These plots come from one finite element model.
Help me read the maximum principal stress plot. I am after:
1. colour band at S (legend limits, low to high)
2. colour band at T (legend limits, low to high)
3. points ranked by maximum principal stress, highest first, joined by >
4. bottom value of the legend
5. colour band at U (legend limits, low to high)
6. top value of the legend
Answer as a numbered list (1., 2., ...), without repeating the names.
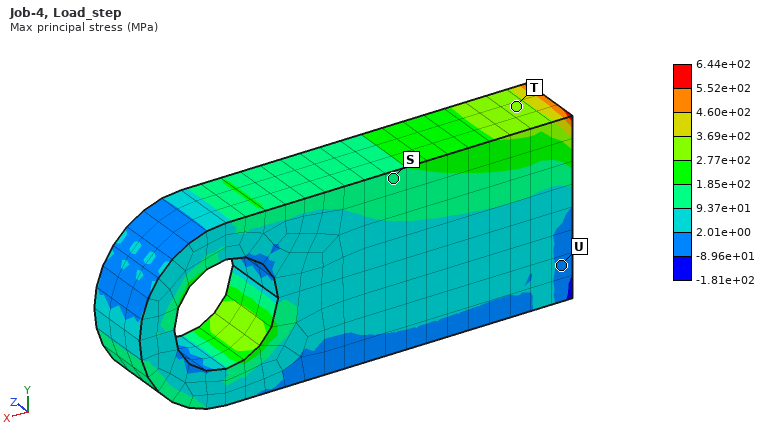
1. 9.37e+01 to 1.85e+02 MPa
2. 2.77e+02 to 3.69e+02 MPa
3. T > S > U
4. -1.81e+02 MPa
5. -8.96e+01 to 2.01e+00 MPa
6. 6.44e+02 MPa
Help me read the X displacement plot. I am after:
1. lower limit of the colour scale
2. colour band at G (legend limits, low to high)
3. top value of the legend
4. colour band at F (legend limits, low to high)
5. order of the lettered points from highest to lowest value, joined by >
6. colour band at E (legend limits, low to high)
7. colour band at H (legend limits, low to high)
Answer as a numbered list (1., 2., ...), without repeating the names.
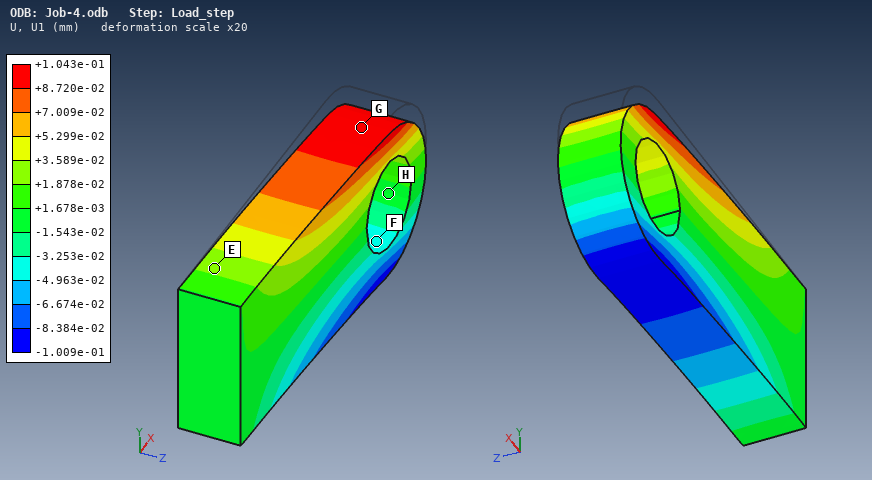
1. -1.009e-01 mm
2. +8.720e-02 to +1.043e-01 mm
3. +1.043e-01 mm
4. -4.963e-02 to -3.253e-02 mm
5. G > E > H > F
6. +1.878e-02 to +3.589e-02 mm
7. -1.543e-02 to +1.678e-03 mm
